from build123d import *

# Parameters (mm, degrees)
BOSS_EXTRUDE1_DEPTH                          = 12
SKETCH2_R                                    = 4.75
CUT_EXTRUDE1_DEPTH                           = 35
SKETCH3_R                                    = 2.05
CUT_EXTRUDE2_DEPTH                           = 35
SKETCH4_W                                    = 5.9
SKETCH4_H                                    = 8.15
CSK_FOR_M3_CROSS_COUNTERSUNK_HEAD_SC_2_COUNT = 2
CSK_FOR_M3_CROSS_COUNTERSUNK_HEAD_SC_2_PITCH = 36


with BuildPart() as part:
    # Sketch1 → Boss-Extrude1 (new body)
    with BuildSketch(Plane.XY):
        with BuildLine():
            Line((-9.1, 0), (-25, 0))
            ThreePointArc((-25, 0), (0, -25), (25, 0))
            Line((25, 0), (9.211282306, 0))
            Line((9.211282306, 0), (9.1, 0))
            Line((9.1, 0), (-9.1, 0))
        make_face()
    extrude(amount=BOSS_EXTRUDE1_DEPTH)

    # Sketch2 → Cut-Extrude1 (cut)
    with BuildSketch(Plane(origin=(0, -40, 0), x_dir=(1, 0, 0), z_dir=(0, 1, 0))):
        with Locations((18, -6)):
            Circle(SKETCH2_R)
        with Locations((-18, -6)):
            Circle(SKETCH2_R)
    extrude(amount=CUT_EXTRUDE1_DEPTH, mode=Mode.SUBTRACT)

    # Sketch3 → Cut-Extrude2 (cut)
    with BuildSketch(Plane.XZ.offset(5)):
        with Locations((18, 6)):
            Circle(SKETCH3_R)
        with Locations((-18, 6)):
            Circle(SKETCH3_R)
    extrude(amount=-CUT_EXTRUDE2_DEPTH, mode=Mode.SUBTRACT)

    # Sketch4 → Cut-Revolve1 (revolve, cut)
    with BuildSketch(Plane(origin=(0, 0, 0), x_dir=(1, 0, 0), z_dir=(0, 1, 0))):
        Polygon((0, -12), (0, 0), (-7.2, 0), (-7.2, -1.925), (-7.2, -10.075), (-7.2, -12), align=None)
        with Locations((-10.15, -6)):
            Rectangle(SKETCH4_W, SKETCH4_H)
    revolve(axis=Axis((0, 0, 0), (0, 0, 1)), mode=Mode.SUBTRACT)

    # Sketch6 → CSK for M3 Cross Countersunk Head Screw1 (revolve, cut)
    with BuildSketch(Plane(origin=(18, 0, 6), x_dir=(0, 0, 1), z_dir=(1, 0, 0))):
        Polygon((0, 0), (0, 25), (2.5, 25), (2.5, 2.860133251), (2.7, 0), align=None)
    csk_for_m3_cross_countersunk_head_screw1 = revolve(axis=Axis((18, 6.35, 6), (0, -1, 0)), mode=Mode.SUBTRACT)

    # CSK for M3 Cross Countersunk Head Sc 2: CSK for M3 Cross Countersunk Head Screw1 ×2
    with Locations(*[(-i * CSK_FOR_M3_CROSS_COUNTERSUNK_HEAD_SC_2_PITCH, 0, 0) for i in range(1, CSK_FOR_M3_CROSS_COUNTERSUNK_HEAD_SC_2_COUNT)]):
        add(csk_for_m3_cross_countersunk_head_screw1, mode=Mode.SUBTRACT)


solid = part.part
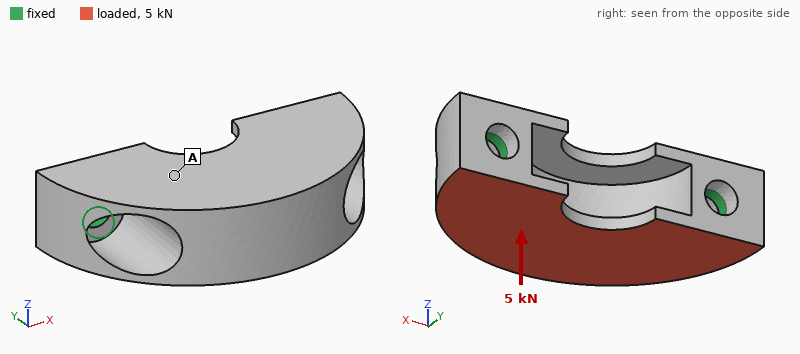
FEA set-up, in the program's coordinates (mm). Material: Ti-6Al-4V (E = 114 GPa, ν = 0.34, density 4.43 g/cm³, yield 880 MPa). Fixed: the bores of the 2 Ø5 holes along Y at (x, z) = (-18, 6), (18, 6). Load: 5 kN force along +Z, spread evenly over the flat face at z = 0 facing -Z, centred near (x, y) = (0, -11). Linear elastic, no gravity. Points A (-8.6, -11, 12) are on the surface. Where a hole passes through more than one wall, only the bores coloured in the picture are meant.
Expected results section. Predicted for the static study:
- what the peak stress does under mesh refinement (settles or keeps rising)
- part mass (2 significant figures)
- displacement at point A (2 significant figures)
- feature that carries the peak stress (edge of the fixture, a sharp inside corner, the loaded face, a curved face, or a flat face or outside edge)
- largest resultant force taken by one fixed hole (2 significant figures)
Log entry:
keeps rising
33 g
0.058 mm
edge of the fixture
2.5 kN
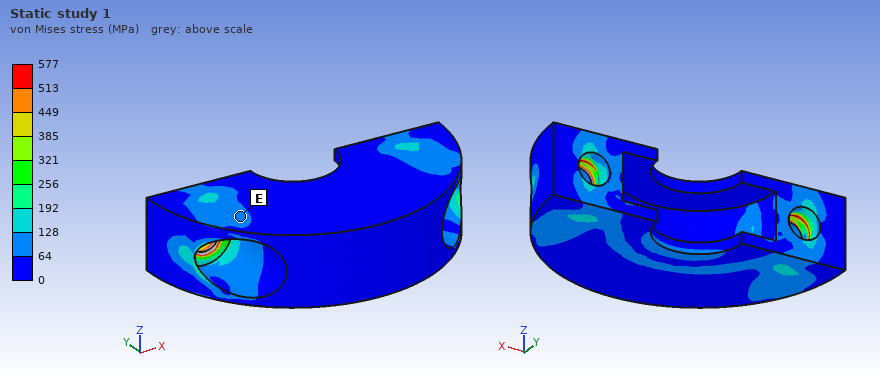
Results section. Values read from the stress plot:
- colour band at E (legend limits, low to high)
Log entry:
64 to 128 MPa
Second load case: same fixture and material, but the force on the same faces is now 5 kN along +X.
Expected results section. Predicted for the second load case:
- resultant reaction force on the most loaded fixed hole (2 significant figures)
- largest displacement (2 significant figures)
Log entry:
2.8 kN
20 µm
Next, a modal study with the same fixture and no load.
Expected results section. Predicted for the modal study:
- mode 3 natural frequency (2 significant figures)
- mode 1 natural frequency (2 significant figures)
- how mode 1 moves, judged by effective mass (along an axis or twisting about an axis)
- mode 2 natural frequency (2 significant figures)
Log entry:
21 kHz
6100 Hz
along Z
21 kHz
